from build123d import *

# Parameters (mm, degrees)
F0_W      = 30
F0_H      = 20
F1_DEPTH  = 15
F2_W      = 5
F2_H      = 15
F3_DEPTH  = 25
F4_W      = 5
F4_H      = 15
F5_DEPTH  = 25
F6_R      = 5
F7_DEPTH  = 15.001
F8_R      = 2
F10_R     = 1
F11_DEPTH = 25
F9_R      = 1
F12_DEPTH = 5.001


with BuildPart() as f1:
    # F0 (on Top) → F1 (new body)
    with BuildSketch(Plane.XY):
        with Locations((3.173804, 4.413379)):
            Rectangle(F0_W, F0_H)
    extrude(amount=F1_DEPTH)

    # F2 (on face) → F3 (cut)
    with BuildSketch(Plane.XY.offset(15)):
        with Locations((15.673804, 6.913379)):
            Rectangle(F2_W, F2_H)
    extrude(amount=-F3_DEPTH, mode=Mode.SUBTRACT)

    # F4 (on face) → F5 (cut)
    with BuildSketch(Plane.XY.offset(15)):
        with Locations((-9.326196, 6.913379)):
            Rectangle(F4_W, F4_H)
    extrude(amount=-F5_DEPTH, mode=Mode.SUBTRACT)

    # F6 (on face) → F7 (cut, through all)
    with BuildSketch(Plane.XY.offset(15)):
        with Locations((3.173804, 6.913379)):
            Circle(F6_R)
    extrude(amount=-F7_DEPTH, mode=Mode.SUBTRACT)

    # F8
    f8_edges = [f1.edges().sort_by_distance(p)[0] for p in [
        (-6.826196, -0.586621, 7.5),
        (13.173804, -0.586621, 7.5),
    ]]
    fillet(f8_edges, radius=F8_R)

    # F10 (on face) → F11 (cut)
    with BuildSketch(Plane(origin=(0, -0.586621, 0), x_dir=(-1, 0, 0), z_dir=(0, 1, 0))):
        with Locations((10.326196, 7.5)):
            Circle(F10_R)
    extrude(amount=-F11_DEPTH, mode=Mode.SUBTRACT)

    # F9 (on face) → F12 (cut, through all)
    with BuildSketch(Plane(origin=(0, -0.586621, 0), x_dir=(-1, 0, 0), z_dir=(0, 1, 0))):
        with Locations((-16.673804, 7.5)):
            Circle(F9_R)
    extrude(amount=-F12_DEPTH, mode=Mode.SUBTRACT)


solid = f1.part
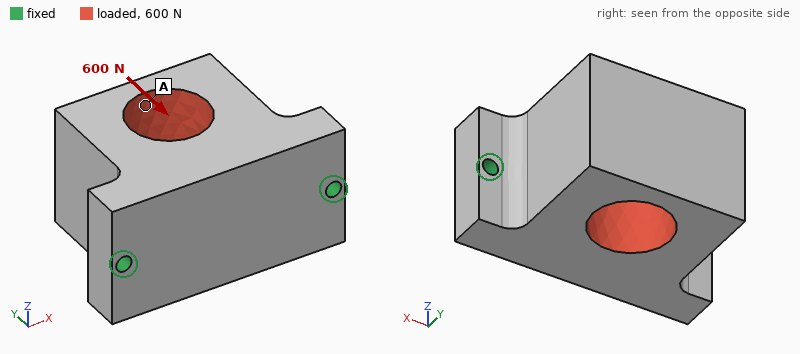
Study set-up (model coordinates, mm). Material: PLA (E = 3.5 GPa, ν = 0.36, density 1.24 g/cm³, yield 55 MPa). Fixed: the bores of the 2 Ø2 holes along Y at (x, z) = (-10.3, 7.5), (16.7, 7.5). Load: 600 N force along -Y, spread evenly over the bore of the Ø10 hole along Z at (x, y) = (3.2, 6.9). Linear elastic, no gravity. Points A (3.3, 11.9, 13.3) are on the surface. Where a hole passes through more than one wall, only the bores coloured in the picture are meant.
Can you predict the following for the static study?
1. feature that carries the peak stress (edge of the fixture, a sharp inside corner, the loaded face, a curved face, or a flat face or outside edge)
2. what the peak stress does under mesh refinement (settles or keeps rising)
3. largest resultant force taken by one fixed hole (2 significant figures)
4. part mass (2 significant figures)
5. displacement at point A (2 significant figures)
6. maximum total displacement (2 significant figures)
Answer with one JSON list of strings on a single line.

["edge of the fixture", "keeps rising", "320 N", "6.9 g", "57 µm", "58 µm"]
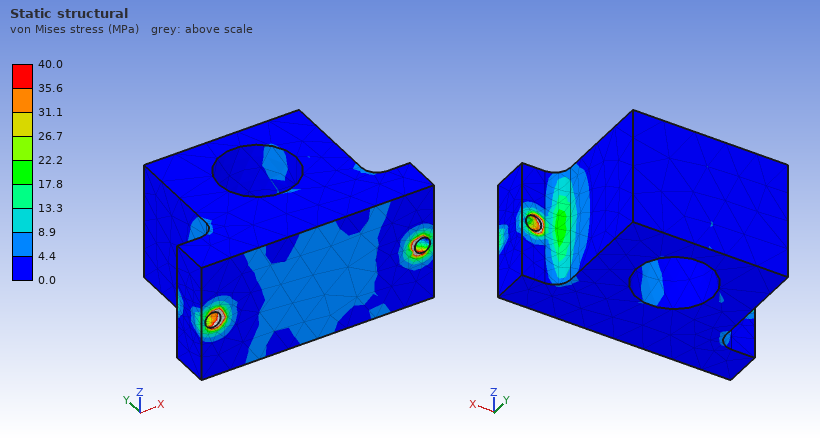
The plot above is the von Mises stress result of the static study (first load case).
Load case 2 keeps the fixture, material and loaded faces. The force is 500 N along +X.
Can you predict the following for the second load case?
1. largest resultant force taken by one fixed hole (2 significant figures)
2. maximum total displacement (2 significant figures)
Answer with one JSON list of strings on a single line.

["320 N", "92 µm"]
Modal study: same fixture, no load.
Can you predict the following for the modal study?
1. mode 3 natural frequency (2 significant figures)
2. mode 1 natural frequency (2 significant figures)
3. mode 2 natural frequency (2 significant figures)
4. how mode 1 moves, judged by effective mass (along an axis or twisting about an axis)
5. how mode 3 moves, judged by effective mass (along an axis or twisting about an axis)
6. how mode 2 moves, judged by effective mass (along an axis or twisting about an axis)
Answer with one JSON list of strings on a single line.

["7000 Hz", "2600 Hz", "6600 Hz", "along Z", "along Y", "along X"]
